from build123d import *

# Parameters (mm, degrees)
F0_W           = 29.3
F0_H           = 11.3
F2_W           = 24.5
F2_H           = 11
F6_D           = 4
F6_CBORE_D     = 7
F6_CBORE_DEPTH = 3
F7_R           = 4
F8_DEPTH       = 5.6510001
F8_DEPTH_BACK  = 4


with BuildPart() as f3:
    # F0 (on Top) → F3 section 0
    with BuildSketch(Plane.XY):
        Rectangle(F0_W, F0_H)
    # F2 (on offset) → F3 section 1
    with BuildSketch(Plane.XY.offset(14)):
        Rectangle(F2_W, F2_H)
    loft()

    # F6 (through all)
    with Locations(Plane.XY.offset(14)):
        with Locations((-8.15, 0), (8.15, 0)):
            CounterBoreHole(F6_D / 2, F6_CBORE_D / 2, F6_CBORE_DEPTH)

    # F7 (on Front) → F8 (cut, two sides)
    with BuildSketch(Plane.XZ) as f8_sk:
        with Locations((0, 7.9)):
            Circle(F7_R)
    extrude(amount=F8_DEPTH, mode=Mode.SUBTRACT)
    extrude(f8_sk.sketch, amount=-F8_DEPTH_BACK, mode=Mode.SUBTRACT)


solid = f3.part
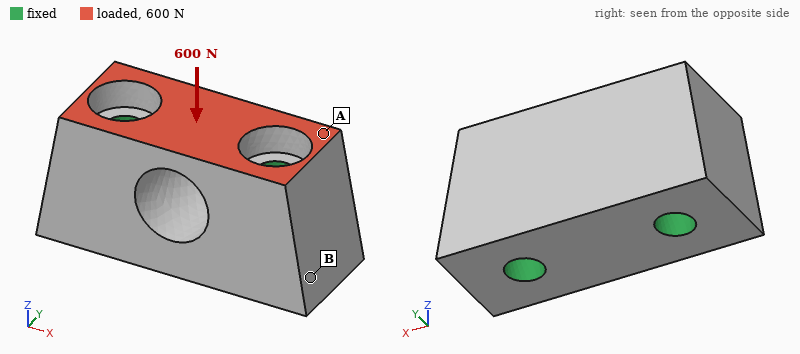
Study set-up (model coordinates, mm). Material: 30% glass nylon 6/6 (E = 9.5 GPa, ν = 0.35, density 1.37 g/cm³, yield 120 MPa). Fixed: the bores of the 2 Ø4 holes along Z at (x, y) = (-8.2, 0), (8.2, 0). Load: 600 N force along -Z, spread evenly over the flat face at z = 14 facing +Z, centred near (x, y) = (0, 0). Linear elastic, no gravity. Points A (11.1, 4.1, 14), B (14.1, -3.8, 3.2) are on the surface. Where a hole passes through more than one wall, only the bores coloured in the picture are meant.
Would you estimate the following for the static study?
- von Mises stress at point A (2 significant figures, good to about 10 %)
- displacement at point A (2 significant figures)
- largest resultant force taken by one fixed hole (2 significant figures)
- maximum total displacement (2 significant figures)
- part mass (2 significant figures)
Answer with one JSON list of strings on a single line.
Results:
["2.9 MPa", "2.6 µm", "310 N", "11 µm", "4.4 g"]
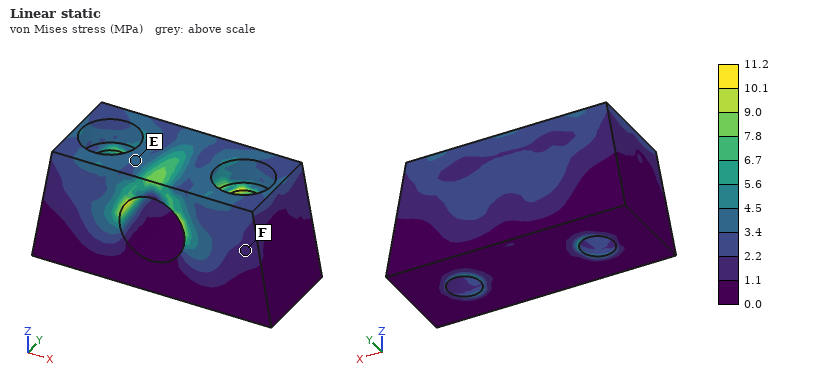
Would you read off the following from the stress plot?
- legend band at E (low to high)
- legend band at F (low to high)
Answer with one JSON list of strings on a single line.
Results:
["3.4 to 4.5 MPa", "1.1 to 2.2 MPa"]
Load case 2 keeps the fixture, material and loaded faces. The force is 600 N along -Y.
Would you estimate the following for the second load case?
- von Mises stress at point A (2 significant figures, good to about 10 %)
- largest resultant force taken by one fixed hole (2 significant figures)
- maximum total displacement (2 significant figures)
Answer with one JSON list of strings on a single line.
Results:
["9.5 MPa", "300 N", "29 µm"]
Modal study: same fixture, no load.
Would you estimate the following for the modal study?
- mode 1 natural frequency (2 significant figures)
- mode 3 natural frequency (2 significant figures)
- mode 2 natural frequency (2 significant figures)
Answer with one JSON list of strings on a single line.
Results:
["34 kHz", "46 kHz", "44 kHz"]
